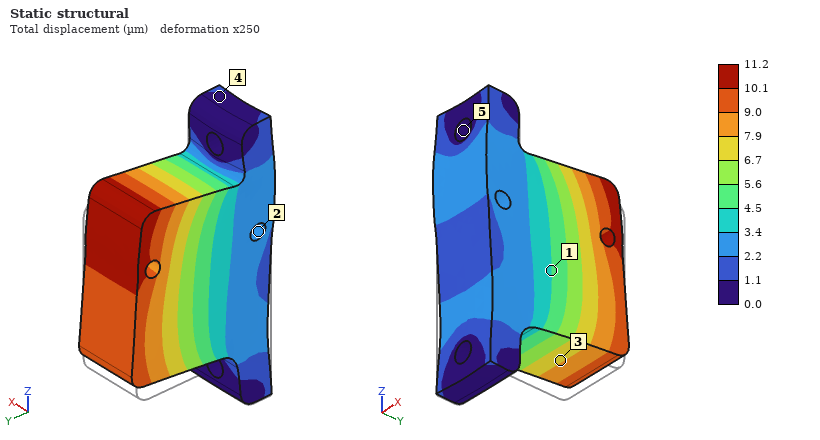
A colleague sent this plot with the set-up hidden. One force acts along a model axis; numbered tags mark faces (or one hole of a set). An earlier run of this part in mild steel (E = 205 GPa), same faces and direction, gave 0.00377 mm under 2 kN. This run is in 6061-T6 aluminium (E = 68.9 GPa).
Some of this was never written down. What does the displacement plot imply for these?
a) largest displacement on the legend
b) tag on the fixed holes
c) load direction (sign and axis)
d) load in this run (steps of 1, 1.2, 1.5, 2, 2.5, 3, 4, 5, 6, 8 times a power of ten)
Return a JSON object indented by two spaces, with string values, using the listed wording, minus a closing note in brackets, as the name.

{
  "largest displacement on the legend": "11.2 µm",
  "tag on the fixed holes": "5",
  "load direction": "+Z",
  "load in this run": "2 kN"
}
